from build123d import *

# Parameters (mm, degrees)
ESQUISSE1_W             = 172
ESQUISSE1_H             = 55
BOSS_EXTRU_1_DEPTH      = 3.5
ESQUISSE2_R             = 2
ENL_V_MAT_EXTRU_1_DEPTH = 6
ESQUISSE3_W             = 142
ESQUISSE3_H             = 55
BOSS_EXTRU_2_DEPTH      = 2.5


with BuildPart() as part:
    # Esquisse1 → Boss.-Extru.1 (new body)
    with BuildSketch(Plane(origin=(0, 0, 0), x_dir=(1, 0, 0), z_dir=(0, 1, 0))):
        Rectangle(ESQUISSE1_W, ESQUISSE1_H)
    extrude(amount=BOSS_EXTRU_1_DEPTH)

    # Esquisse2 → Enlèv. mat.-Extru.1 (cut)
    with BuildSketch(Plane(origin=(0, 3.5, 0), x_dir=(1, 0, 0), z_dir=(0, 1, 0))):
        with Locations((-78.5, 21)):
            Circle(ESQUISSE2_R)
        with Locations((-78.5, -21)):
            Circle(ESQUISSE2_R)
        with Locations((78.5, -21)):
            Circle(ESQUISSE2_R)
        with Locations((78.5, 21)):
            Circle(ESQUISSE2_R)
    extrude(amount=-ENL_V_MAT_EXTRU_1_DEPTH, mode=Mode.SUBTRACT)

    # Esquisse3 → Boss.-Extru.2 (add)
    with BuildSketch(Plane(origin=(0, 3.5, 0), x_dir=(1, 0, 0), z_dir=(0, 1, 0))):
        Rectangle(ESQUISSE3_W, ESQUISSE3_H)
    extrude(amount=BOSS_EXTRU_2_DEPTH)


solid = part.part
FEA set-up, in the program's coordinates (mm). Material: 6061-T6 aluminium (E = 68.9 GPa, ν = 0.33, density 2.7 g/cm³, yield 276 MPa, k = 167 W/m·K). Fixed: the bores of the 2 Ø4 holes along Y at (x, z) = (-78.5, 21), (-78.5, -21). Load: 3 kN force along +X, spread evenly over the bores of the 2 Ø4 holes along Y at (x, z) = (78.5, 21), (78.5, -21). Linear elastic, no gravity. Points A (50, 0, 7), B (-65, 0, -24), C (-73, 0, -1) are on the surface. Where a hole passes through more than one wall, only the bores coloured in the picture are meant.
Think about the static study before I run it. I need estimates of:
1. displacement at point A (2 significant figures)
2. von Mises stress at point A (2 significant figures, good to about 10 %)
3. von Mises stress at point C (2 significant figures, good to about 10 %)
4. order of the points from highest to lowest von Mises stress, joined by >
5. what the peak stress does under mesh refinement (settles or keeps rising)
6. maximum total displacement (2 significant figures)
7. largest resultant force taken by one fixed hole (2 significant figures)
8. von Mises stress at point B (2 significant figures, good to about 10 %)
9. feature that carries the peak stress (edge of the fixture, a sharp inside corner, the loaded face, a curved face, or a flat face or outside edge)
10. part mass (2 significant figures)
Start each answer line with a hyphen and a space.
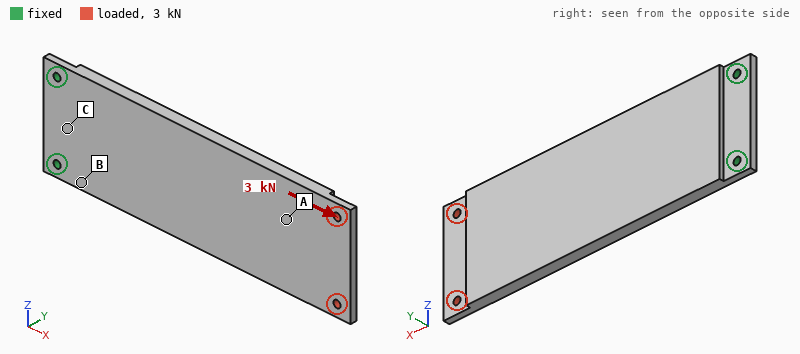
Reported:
- 0.40 mm
- 18 MPa
- 7.6 MPa
- B > A > C
- keeps rising
- 0.66 mm
- 1.5 kN
- 27 MPa
- edge of the fixture
- 140 g
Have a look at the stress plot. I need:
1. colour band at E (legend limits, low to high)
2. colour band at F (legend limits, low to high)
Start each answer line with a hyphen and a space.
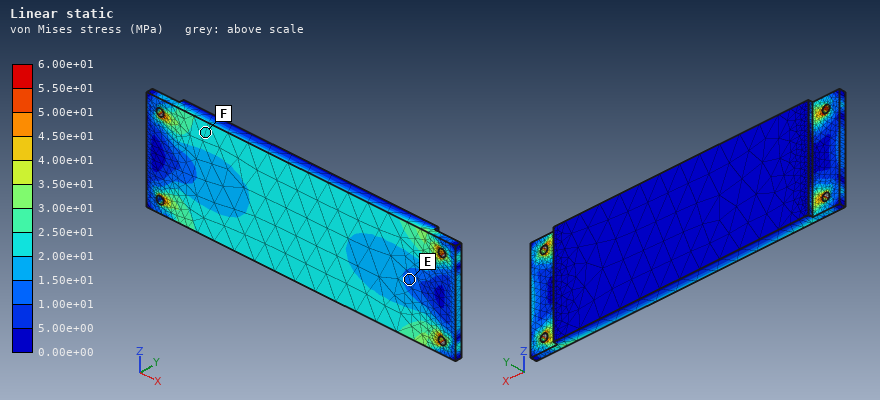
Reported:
- 1.00e+01 to 1.50e+01 MPa
- 2.00e+01 to 2.50e+01 MPa
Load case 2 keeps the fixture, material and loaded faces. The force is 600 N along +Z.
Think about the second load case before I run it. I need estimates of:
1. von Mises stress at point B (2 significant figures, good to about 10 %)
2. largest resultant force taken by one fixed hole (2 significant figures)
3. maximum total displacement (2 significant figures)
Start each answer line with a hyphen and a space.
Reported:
- 42 MPa
- 2.2 kN
- 0.22 mm
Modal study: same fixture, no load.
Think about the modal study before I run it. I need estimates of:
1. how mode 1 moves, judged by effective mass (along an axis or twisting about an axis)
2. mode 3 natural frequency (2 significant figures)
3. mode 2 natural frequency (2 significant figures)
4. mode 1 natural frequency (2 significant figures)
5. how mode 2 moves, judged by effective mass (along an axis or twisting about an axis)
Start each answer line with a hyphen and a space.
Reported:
- along Y
- 1000 Hz
- 1000 Hz
- 130 Hz
- along Y
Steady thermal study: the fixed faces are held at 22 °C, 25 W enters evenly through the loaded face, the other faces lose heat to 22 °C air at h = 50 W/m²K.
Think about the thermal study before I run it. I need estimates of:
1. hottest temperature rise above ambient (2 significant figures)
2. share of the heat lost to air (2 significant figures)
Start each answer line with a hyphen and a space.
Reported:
- 47 K
- 71 %
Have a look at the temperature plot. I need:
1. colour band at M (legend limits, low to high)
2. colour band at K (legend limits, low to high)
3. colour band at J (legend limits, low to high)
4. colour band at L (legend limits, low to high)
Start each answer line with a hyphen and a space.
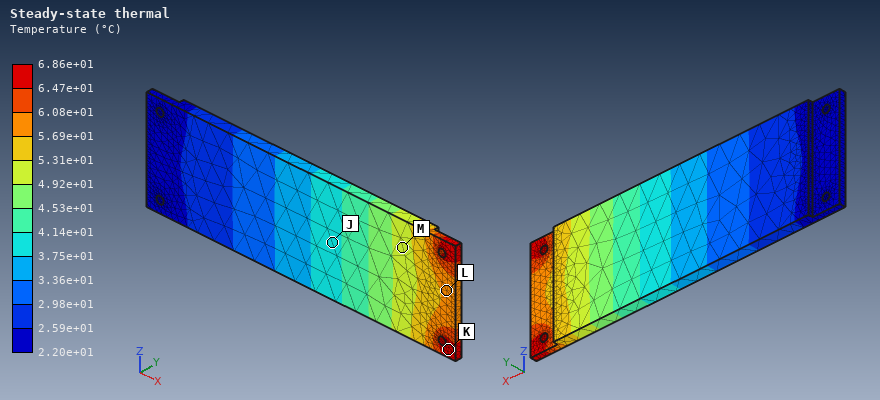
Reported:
- 4.92e+01 to 5.31e+01 °C
- 6.47e+01 to 6.86e+01 °C
- 3.75e+01 to 4.14e+01 °C
- 5.69e+01 to 6.08e+01 °C
